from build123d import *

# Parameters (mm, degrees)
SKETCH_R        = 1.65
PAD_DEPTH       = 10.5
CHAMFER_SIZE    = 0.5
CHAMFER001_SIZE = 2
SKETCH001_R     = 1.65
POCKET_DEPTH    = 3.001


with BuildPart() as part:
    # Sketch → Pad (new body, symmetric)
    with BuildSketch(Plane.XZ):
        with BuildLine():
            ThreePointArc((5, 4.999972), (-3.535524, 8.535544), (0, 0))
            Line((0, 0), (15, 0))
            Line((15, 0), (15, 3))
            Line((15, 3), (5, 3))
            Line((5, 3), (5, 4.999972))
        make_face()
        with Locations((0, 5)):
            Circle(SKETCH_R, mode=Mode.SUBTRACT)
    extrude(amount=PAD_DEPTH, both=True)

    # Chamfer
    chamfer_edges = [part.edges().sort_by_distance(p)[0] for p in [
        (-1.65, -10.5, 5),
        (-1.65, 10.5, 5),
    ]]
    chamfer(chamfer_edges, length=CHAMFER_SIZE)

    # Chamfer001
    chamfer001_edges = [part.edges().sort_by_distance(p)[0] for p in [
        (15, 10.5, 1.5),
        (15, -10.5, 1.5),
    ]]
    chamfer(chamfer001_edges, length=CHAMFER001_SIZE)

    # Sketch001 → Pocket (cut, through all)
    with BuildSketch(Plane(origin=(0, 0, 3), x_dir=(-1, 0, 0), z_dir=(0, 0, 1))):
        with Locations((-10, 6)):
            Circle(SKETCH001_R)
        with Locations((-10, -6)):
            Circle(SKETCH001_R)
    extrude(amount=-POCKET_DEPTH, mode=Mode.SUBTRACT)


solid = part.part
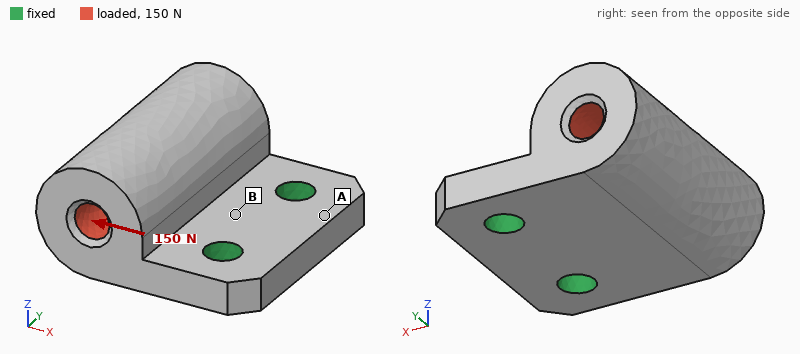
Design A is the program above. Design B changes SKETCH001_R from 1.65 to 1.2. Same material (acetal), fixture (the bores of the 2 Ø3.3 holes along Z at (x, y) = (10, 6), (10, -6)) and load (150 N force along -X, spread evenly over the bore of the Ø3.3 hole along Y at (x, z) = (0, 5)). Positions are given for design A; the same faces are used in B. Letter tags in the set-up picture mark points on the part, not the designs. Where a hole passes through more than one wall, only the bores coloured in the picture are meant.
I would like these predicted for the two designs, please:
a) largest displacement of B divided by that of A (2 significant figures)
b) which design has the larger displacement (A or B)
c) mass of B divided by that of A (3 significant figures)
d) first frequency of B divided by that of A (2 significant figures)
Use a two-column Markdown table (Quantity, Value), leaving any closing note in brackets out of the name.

| Quantity | Value |
|---|---|
| largest displacement of B divided by that of A | 1.1 |
| which design has the larger displacement | B |
| mass of B divided by that of A | 1.01 |
| first frequency of B divided by that of A | 0.91 |
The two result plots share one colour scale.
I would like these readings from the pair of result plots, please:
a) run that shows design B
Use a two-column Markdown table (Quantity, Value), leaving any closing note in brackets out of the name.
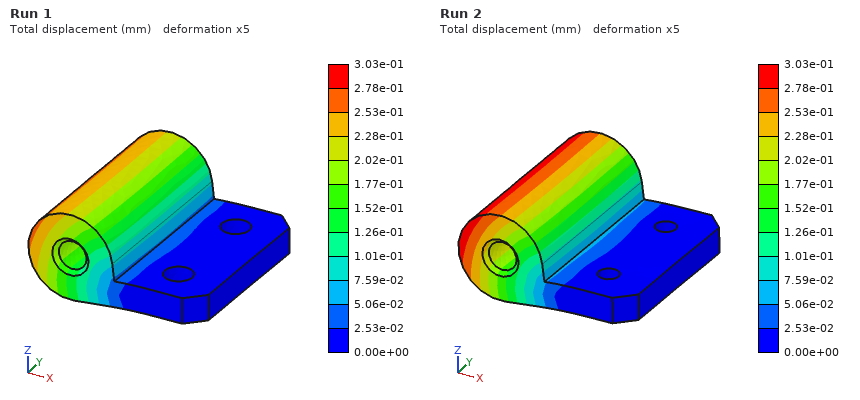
| Quantity | Value |
|---|---|
| run that shows design B | Run 2 |
